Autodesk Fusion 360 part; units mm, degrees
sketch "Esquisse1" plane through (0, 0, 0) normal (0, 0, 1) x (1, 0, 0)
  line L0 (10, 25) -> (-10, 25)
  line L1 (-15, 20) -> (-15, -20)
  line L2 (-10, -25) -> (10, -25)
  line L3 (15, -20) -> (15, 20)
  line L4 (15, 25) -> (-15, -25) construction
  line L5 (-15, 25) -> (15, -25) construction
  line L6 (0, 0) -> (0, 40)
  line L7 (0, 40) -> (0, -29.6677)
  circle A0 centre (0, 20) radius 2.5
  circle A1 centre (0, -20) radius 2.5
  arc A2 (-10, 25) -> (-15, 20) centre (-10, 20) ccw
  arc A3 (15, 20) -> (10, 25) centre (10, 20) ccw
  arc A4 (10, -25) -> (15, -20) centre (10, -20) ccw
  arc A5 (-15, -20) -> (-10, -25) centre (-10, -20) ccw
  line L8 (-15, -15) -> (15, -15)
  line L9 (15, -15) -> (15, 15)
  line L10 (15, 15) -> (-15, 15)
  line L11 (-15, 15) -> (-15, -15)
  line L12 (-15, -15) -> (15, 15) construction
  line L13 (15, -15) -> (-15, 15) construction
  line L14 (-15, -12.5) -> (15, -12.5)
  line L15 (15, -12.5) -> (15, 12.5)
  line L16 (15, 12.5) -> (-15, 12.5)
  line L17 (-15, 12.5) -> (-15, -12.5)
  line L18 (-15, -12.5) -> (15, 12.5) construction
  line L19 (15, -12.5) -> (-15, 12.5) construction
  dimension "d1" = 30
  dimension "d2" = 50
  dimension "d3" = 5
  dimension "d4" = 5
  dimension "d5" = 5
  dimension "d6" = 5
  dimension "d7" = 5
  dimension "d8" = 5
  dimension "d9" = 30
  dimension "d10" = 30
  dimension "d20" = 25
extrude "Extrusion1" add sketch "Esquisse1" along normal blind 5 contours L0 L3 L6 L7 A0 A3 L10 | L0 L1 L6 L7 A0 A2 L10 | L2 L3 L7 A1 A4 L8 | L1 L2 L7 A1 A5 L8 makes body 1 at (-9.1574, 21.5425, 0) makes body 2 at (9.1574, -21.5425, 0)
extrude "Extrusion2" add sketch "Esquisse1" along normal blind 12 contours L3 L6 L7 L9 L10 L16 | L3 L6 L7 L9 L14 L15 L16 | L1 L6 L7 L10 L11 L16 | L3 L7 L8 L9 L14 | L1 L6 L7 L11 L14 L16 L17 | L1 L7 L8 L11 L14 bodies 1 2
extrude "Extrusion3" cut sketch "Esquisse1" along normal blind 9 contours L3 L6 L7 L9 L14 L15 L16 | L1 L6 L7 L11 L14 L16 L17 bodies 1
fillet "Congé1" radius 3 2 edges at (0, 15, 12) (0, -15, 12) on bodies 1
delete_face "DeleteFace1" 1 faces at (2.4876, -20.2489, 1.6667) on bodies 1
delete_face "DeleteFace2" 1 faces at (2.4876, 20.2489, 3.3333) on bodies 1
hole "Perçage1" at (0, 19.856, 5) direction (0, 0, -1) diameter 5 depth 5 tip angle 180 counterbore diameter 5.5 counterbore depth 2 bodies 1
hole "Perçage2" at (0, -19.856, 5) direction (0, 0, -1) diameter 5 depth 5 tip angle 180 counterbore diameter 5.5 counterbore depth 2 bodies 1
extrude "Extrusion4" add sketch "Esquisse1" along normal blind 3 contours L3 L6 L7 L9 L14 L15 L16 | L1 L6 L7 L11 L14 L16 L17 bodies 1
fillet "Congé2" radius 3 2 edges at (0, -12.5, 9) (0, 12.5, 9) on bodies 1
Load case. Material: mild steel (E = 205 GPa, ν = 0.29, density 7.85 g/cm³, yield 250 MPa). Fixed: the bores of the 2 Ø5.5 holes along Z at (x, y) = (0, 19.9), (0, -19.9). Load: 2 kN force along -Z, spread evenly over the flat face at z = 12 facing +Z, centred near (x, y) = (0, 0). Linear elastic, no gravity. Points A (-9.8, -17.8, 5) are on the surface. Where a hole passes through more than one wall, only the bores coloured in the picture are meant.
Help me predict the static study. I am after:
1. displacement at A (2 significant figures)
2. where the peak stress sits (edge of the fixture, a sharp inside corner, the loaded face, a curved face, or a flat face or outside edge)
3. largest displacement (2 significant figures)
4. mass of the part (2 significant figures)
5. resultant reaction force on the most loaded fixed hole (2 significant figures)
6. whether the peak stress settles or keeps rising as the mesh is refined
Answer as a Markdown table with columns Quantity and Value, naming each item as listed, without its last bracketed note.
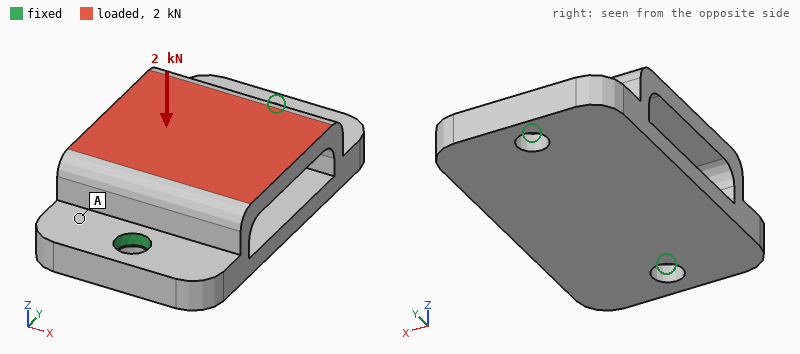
| Quantity | Value |
|---|---|
| displacement at A | 2.2 µm |
| where the peak stress sits | edge of the fixture |
| largest displacement | 13 µm |
| mass of the part | 70 g |
| resultant reaction force on the most loaded fixed hole | 1.1 kN |
| whether the peak stress settles or keeps rising as the mesh is refined | keeps rising |
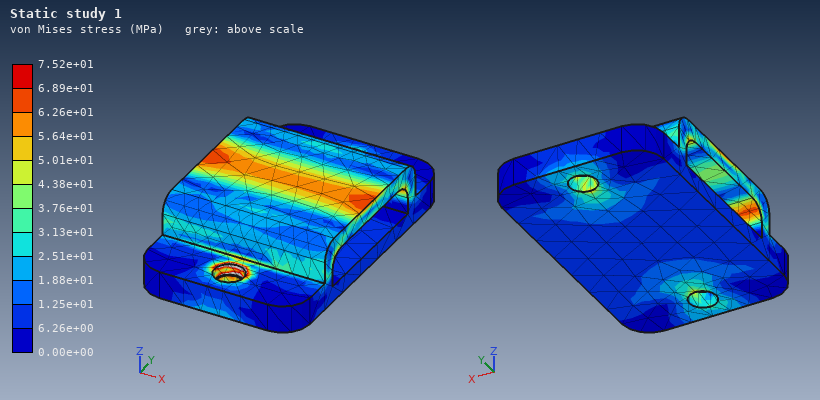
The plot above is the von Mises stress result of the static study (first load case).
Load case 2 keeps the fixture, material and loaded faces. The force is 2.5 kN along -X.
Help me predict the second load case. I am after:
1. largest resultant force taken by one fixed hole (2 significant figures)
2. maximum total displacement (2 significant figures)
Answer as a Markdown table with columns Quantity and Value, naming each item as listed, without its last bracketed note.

| Quantity | Value |
|---|---|
| largest resultant force taken by one fixed hole | 1.3 kN |
| maximum total displacement | 30 µm |
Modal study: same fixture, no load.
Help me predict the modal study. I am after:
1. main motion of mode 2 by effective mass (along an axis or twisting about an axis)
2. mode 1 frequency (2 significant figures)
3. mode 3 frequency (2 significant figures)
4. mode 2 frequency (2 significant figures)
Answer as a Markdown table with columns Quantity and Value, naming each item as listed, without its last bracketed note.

| Quantity | Value |
|---|---|
| main motion of mode 2 by effective mass | along Z |
| mode 1 frequency | 7500 Hz |
| mode 3 frequency | 15 kHz |
| mode 2 frequency | 13 kHz |
